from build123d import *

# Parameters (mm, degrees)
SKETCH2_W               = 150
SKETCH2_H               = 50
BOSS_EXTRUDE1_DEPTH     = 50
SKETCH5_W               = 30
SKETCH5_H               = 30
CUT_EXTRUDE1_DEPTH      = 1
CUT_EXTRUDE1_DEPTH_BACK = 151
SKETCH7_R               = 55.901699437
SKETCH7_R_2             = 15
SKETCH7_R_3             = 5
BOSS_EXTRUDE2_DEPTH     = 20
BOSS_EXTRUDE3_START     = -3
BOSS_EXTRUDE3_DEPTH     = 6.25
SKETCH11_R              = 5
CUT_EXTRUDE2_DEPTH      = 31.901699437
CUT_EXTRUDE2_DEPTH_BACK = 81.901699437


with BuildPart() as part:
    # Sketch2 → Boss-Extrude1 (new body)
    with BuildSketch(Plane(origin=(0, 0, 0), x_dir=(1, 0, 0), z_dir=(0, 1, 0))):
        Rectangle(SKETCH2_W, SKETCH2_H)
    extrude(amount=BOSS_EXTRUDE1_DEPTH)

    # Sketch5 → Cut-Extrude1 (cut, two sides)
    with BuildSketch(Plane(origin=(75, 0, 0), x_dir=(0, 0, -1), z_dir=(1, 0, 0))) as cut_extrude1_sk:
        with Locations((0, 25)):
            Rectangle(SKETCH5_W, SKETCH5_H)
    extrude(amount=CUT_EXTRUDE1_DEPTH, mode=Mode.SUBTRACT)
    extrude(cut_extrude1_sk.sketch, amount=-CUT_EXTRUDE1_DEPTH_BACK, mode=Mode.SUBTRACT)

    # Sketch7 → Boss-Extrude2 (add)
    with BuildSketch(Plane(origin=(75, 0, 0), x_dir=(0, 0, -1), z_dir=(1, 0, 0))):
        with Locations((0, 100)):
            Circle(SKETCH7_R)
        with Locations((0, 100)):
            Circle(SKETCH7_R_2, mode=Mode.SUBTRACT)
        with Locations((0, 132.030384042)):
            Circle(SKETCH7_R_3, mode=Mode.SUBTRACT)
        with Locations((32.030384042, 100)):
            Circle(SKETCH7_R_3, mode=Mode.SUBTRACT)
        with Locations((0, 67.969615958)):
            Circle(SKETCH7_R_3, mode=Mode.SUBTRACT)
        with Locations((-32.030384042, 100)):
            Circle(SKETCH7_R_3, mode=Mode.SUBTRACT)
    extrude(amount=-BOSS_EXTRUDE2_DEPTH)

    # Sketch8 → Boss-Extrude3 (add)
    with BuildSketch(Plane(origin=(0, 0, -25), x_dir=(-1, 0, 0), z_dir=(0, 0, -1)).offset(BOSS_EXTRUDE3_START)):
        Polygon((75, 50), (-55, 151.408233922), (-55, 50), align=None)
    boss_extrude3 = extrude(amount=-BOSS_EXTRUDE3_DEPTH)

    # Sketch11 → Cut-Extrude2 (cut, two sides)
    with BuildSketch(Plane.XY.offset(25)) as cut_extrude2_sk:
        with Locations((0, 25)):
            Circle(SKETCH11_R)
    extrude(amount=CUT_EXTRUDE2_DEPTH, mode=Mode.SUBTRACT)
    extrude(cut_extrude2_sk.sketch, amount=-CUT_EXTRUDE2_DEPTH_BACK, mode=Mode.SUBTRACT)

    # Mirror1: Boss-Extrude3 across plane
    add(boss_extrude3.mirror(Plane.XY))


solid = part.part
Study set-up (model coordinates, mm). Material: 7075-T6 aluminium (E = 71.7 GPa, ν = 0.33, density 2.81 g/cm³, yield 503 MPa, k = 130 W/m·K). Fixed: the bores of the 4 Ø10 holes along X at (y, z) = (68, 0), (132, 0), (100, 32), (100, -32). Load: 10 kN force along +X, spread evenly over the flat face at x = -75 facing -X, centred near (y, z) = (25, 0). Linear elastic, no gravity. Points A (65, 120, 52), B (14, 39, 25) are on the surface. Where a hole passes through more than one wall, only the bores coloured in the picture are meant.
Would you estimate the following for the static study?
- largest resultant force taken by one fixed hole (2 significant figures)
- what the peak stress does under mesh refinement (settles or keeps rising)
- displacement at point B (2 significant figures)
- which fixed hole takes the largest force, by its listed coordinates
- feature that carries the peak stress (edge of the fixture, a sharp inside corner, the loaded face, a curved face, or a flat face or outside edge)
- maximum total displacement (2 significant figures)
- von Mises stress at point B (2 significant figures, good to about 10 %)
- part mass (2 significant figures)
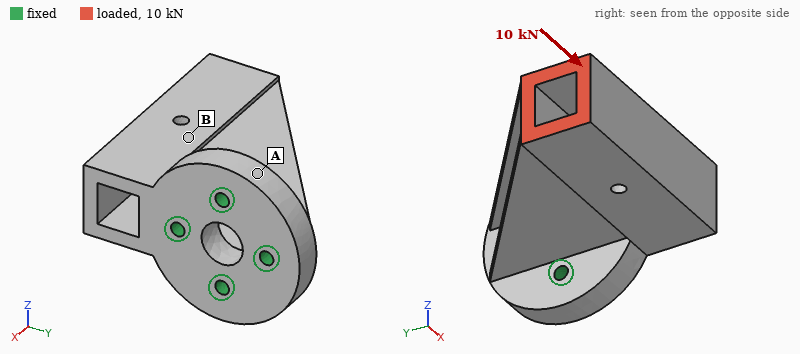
13 kN
keeps rising
0.041 mm
(68, 0)
edge of the fixture
0.10 mm
9.5 MPa
1.4 kg
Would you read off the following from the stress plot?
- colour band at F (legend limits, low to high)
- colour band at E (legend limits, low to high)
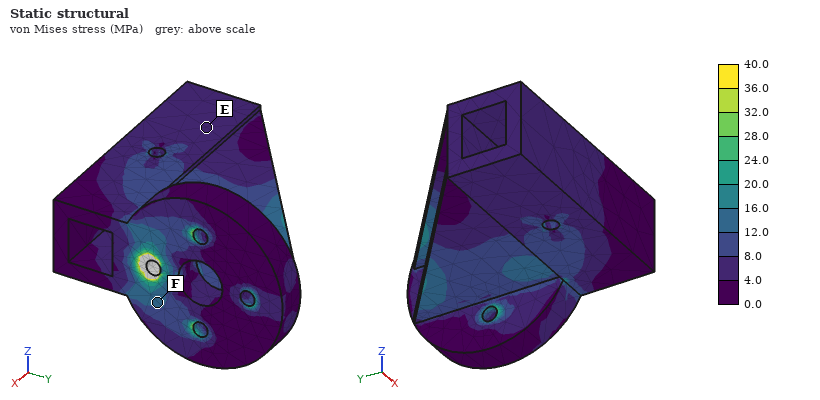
12.0 to 16.0 MPa
4.0 to 8.0 MPa
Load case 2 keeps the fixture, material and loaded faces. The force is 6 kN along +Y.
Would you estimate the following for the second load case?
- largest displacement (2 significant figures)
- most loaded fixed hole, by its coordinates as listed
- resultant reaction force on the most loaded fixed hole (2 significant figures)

0.16 mm
(68, 0)
11 kN
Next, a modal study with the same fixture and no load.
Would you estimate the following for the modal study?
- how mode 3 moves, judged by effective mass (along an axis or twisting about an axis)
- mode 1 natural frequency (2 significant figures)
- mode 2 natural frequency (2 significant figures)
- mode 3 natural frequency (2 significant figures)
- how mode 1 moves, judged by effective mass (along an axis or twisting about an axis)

twisting about X
1100 Hz
1900 Hz
2600 Hz
along Z
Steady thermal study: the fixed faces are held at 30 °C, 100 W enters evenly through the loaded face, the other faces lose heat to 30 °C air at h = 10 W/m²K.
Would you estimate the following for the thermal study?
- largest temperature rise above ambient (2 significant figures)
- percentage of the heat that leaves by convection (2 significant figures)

58 K
19 %
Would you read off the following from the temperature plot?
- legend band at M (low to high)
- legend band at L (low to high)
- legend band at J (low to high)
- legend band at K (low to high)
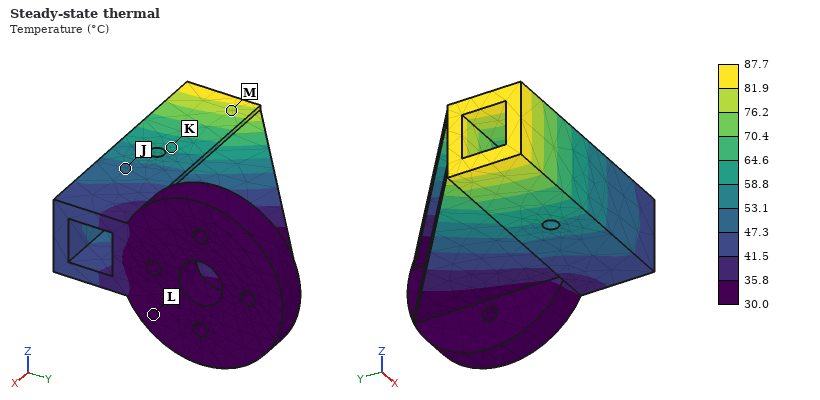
76.2 to 81.9 °C
30.0 to 35.8 °C
47.3 to 53.1 °C
58.8 to 64.6 °C
